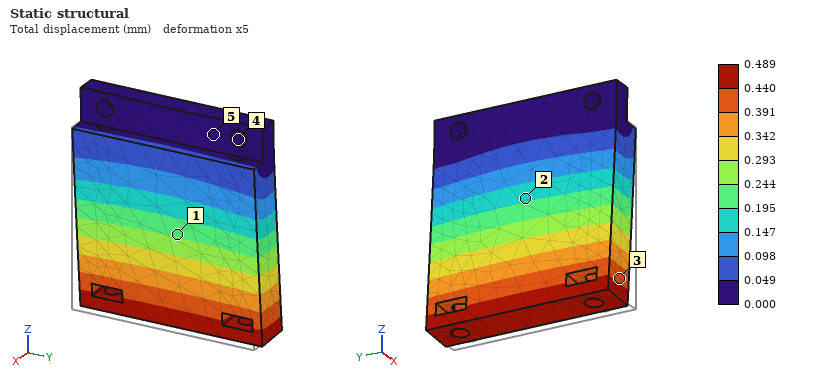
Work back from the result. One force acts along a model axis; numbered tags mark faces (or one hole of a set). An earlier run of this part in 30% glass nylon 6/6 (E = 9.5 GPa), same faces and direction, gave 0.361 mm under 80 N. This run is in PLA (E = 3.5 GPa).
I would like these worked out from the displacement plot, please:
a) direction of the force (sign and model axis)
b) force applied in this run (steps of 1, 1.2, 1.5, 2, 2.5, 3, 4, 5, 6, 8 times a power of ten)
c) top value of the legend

-X
40 N
0.489 mm
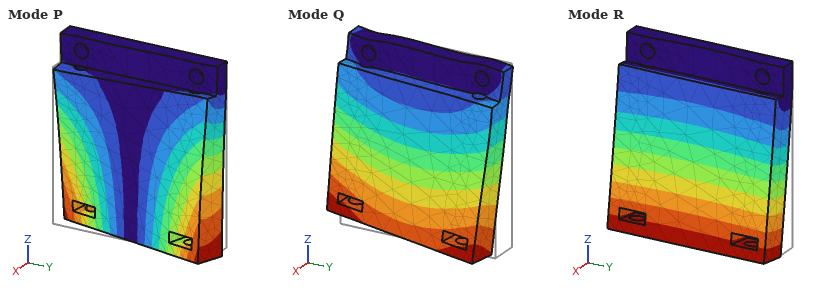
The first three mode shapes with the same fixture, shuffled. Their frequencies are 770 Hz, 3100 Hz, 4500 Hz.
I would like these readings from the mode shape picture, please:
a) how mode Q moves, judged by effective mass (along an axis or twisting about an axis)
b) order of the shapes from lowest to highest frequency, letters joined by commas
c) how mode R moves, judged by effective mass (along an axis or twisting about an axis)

along Y
R, P, Q
along X
